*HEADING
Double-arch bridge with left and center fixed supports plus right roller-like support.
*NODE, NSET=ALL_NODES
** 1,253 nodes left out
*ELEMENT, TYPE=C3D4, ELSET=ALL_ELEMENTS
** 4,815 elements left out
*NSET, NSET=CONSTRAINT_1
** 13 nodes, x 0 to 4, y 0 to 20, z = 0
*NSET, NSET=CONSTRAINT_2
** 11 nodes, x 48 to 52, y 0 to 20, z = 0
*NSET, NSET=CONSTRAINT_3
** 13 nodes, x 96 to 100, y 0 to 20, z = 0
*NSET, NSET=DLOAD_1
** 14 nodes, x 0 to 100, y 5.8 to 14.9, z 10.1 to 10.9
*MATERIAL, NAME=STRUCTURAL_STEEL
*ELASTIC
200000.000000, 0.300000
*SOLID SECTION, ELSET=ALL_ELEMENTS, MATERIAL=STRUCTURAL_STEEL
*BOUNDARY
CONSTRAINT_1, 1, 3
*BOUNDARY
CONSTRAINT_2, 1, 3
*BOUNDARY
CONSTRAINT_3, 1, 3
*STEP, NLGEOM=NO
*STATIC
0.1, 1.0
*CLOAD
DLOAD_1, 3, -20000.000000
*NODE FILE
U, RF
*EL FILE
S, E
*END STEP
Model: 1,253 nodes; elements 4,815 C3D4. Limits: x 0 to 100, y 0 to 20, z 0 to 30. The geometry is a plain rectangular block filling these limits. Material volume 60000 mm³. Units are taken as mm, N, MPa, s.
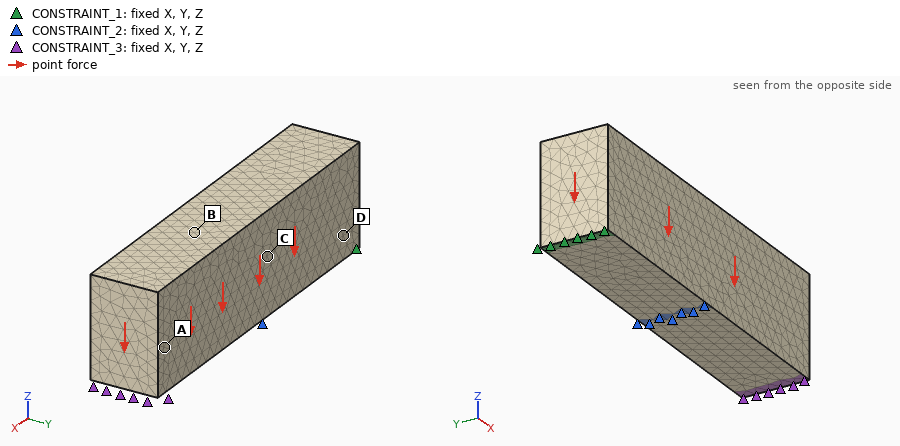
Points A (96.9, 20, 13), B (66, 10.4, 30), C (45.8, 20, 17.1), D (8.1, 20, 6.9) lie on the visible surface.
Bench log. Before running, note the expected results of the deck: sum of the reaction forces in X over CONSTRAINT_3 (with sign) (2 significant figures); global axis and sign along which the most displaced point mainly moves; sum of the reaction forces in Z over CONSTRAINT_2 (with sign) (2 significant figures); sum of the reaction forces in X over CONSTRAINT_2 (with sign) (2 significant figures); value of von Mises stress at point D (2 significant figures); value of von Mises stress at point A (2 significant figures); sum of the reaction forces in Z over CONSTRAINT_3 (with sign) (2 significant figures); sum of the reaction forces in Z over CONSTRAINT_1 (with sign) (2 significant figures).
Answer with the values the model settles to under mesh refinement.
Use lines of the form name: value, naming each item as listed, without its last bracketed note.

sum of the reaction forces in X over CONSTRAINT_3 (with sign): -19000 N
global axis and sign along which the most displaced point mainly moves: -Z
sum of the reaction forces in Z over CONSTRAINT_2 (with sign): 91000 N
sum of the reaction forces in X over CONSTRAINT_2 (with sign): 6000 N
value of von Mises stress at point D: 220 MPa
value of von Mises stress at point A: 370 MPa
sum of the reaction forces in Z over CONSTRAINT_3 (with sign): 96000 N
sum of the reaction forces in Z over CONSTRAINT_1 (with sign): 92000 N
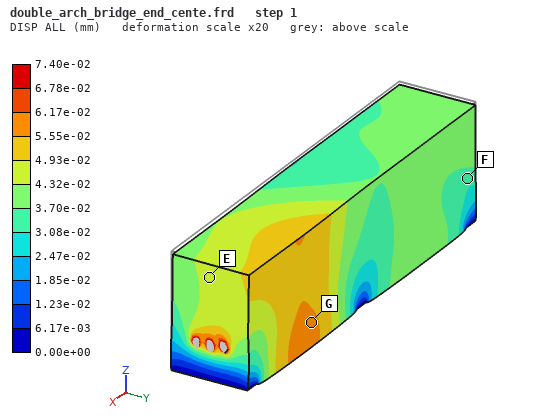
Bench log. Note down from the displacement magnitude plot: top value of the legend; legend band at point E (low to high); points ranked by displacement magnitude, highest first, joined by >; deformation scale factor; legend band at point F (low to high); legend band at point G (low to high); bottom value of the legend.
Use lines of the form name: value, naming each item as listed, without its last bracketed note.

top value of the legend: 7.40e-02 mm
legend band at point E: 4.32e-02 to 4.93e-02 mm
points ranked by displacement magnitude, highest first, joined by >: G > E > F
deformation scale factor: 20
legend band at point F: 3.08e-02 to 3.70e-02 mm
legend band at point G: 5.55e-02 to 6.17e-02 mm
bottom value of the legend: 0.00e+00 mm
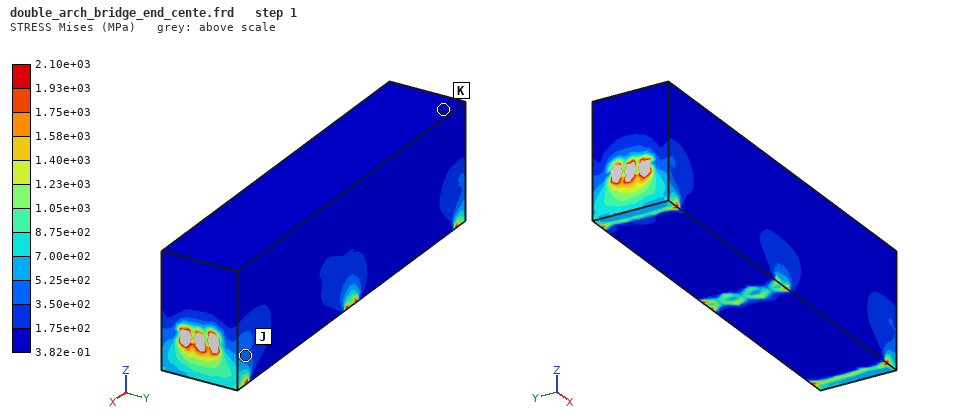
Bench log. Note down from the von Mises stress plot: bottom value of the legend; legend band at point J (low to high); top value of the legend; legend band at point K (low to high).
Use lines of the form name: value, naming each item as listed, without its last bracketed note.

bottom value of the legend: 3.82e-01 MPa
legend band at point J: 3.50e+02 to 5.25e+02 MPa
top value of the legend: 2.10e+03 MPa
legend band at point K: 3.82e-01 to 1.75e+02 MPa
